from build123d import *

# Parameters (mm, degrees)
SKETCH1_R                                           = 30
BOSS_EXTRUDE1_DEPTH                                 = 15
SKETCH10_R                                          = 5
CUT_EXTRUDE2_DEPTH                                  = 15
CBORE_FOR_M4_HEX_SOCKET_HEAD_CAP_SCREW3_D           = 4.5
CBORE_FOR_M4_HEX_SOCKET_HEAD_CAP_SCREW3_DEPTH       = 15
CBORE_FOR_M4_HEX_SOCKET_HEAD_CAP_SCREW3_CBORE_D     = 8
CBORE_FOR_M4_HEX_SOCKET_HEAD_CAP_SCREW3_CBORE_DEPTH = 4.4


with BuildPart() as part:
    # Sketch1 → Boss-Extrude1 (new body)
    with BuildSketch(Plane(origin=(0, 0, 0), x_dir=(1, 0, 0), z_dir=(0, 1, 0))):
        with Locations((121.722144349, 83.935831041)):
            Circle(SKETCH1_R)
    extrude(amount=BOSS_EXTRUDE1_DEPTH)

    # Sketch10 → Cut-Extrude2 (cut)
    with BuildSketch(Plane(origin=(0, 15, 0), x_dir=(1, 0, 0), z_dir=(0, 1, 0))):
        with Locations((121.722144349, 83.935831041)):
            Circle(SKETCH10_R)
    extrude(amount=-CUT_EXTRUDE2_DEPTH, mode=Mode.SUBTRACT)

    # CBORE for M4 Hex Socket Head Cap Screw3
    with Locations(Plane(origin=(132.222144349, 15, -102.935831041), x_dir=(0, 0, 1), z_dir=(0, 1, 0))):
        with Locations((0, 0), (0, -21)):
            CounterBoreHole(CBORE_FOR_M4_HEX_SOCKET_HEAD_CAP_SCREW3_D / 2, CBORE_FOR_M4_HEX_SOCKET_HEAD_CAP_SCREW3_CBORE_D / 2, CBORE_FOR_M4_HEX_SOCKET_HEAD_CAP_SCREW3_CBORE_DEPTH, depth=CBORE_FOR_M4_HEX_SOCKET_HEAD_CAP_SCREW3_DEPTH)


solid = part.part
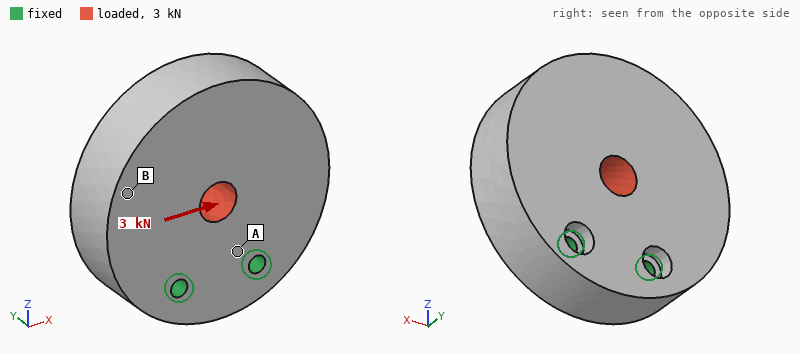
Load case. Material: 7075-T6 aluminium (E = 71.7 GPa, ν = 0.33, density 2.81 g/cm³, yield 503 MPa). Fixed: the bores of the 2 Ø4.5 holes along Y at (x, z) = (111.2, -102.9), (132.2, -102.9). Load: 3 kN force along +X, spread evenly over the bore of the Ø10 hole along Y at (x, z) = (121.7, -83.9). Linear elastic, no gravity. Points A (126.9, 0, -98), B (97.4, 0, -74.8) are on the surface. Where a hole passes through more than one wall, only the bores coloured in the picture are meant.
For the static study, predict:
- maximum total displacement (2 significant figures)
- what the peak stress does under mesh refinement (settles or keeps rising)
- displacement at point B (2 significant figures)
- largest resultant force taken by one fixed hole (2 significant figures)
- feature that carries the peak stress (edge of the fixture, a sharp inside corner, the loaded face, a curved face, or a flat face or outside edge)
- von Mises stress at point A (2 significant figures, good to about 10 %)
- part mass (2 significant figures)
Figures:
15 µm
keeps rising
12 µm
2.8 kN
edge of the fixture
17 MPa
110 g
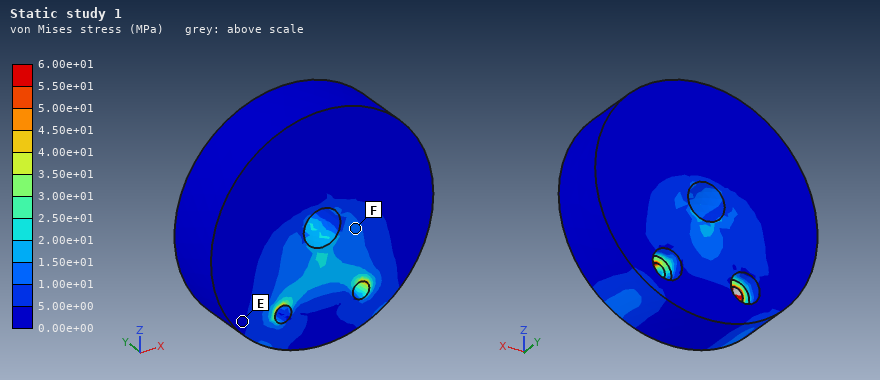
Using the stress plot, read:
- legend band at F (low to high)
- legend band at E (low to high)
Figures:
1.00e+01 to 1.50e+01 MPa
0.00e+00 to 5.00e+00 MPa
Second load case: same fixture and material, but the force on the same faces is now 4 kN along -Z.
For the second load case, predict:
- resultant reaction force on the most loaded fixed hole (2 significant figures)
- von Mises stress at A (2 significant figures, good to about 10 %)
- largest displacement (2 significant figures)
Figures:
2.0 kN
5.9 MPa
8.2 µm
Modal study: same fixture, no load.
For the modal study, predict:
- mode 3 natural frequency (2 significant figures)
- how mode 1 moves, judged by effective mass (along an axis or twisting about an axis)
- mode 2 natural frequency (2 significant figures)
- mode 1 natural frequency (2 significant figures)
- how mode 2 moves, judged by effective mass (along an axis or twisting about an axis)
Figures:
8400 Hz
along Y
7200 Hz
3800 Hz
along X
